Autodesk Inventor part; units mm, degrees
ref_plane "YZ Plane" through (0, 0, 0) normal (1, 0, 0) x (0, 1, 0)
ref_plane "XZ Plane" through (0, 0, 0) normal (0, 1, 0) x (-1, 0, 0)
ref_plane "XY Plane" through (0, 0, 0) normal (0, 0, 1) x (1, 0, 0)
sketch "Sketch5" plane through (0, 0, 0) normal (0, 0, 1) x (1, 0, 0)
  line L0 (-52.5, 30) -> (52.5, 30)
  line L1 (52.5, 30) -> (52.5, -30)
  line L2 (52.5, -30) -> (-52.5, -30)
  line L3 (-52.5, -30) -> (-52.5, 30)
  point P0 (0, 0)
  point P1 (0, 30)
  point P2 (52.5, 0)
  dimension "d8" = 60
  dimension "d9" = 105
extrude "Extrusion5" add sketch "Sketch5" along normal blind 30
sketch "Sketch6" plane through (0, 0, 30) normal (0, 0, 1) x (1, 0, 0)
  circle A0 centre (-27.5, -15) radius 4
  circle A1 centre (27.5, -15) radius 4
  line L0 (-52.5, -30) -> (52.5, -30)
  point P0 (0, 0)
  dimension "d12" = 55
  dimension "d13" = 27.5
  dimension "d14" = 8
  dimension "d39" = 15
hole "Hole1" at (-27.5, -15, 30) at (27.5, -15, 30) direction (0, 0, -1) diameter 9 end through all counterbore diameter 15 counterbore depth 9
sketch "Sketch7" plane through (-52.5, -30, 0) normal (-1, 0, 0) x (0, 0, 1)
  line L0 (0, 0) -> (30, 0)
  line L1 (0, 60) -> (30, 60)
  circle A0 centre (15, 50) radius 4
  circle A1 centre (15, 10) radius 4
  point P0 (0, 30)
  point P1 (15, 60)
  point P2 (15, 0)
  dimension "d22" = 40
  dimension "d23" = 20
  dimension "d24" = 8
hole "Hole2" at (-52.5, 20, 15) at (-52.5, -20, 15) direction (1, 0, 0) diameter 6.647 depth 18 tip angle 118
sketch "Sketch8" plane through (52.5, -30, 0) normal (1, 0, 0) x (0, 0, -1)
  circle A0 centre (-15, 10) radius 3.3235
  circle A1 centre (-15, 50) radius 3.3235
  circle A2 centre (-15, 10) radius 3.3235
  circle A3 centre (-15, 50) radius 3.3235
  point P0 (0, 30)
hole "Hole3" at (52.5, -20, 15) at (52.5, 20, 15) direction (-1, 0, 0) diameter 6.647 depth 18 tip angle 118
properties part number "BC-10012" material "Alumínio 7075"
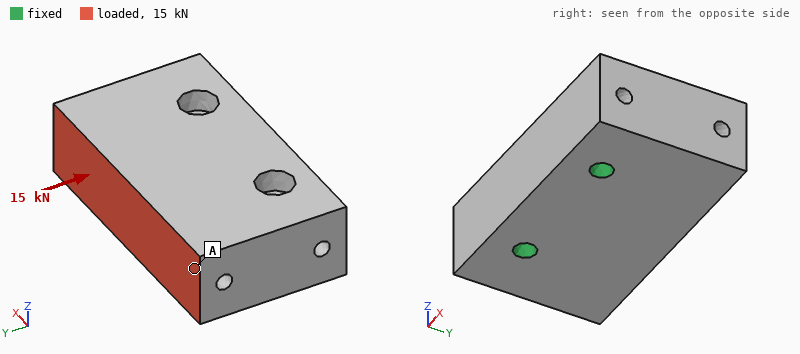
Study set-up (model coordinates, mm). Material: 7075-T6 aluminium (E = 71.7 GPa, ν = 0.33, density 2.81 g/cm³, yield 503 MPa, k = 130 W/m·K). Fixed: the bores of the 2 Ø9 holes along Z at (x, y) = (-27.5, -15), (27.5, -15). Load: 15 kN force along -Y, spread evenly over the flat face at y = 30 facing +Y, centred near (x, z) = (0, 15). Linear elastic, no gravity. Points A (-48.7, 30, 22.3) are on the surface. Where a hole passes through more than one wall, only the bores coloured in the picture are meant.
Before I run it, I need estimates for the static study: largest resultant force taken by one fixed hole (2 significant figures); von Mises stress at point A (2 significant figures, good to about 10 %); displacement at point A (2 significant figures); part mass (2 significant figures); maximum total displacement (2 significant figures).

7.5 kN
5.1 MPa
9.2 µm
510 g
10.0 µm
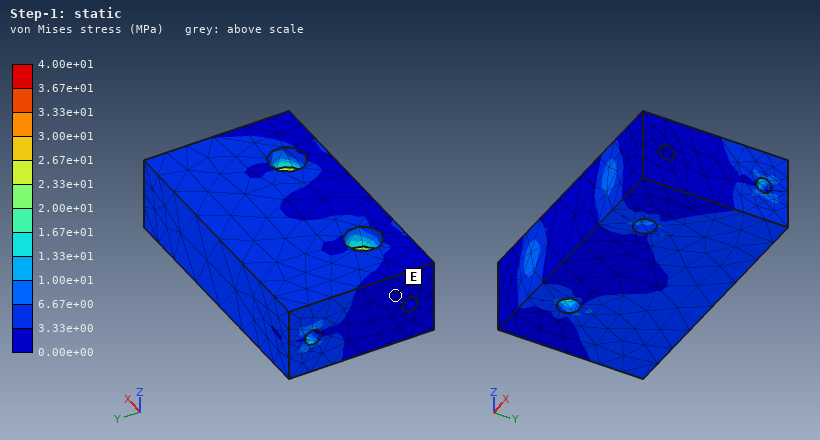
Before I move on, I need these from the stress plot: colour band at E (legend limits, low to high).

0.00e+00 to 3.33e+00 MPa
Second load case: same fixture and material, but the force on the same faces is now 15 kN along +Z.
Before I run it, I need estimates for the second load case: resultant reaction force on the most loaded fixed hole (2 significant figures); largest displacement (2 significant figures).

7.5 kN
94 µm
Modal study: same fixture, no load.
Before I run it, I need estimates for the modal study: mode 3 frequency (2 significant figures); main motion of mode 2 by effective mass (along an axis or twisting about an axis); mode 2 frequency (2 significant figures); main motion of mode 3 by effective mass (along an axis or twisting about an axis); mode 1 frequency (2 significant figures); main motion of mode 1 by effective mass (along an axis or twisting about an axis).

10 kHz
twisting about Y
8700 Hz
along X
5700 Hz
along Z
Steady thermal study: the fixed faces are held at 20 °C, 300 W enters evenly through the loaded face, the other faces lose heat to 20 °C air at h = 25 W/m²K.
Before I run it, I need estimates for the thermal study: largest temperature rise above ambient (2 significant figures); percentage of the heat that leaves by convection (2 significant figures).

41 K
3.1 %
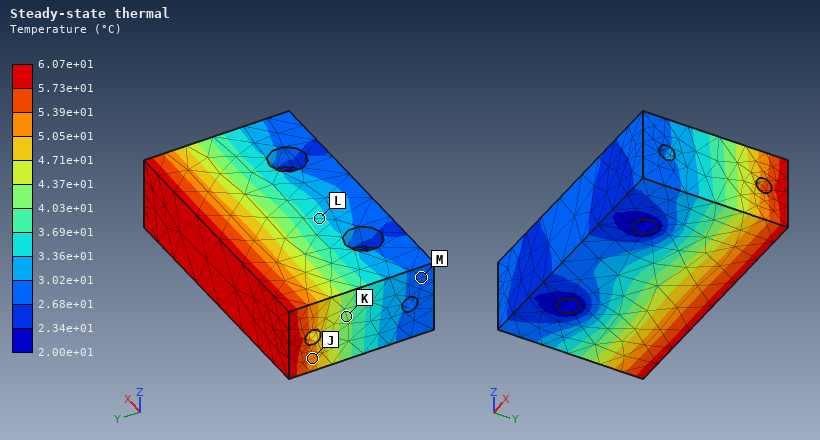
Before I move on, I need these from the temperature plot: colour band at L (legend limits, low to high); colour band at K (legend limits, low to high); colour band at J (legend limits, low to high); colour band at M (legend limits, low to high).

3.36e+01 to 3.69e+01 °C
4.03e+01 to 4.37e+01 °C
5.05e+01 to 5.39e+01 °C
2.68e+01 to 3.02e+01 °C
